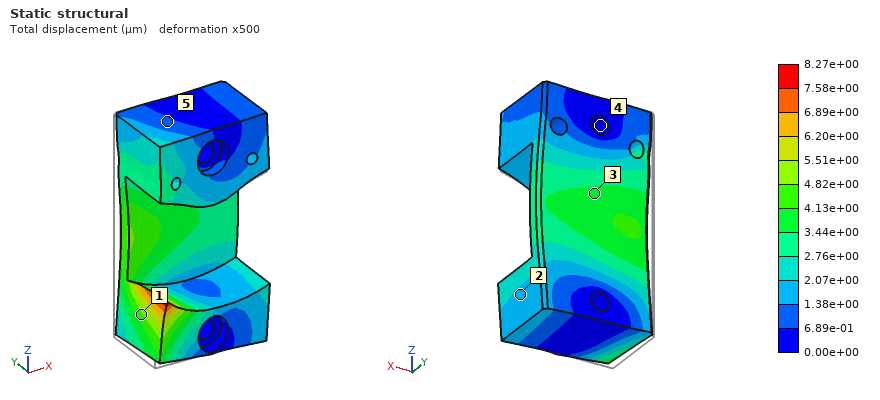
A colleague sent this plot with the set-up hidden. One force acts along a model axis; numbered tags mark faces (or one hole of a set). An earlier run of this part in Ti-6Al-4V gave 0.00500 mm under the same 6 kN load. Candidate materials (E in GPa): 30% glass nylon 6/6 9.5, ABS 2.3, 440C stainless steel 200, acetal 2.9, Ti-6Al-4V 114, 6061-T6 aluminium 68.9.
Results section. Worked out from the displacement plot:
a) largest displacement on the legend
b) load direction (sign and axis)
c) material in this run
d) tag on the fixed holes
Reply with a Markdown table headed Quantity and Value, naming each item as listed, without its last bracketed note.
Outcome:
| Quantity | Value |
|---|---|
| largest displacement on the legend | 8.27e+00 µm |
| load direction | +X |
| material in this run | 6061-T6 aluminium |
| tag on the fixed holes | 4 |
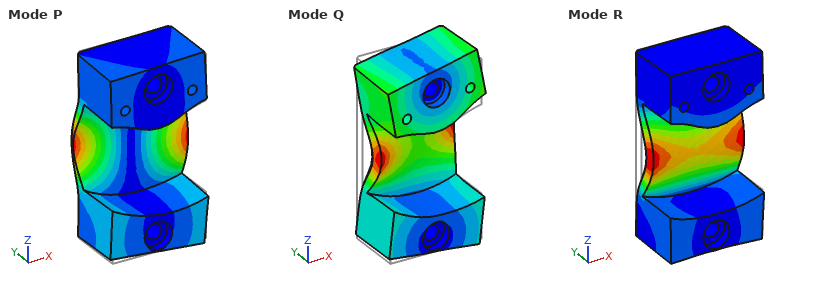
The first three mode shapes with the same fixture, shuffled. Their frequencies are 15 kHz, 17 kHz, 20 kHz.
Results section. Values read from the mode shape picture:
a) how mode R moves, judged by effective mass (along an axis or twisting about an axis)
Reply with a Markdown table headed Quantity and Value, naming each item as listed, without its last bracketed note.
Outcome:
| Quantity | Value |
|---|---|
| how mode R moves, judged by effective mass | along Y |
